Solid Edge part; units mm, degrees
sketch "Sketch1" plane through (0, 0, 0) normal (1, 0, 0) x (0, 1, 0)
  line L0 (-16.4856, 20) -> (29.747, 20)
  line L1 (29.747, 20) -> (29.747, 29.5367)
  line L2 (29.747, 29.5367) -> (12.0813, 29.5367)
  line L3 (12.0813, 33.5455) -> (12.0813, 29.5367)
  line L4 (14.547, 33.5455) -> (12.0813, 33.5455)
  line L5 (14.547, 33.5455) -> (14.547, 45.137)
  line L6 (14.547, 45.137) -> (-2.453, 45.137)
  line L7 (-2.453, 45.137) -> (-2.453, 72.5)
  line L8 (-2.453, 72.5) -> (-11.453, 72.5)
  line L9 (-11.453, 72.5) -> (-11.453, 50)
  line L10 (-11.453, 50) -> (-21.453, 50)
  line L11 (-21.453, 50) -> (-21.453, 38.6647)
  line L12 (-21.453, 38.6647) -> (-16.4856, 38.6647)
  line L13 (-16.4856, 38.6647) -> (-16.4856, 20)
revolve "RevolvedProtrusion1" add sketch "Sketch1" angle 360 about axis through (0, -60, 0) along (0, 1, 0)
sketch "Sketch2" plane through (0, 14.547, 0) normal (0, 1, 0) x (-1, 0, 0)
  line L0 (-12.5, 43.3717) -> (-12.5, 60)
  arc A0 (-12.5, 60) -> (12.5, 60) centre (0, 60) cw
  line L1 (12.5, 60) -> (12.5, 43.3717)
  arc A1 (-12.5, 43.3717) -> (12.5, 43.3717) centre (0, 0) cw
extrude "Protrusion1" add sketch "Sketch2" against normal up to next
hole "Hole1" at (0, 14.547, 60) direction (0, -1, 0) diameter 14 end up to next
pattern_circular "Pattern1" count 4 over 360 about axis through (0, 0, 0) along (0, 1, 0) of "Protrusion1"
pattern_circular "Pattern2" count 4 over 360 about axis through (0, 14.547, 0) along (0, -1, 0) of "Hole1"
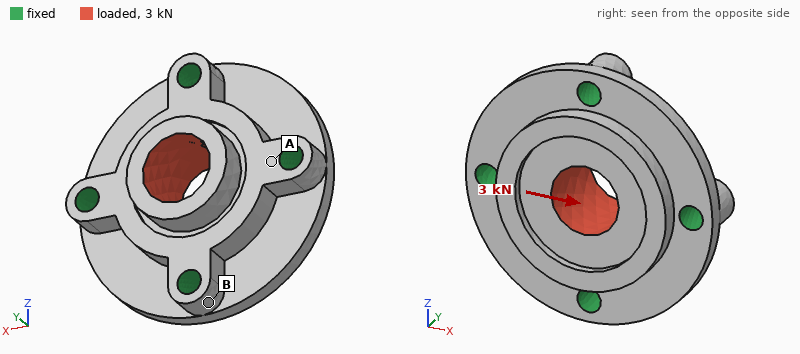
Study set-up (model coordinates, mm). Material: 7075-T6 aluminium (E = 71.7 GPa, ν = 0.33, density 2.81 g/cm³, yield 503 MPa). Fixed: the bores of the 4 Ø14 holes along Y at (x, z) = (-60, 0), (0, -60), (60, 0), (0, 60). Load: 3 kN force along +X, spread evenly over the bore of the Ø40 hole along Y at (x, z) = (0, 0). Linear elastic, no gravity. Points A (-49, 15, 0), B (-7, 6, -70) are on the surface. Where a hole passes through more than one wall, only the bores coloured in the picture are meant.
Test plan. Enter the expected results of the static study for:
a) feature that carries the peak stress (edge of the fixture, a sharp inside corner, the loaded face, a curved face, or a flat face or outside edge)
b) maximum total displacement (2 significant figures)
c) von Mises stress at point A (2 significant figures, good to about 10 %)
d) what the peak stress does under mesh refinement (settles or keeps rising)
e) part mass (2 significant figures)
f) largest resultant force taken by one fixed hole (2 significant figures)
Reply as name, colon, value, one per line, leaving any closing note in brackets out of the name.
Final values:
feature that carries the peak stress: edge of the fixture
maximum total displacement: 1.8 µm
von Mises stress at point A: 1.2 MPa
what the peak stress does under mesh refinement: keeps rising
part mass: 900 g
largest resultant force taken by one fixed hole: 1.0 kN
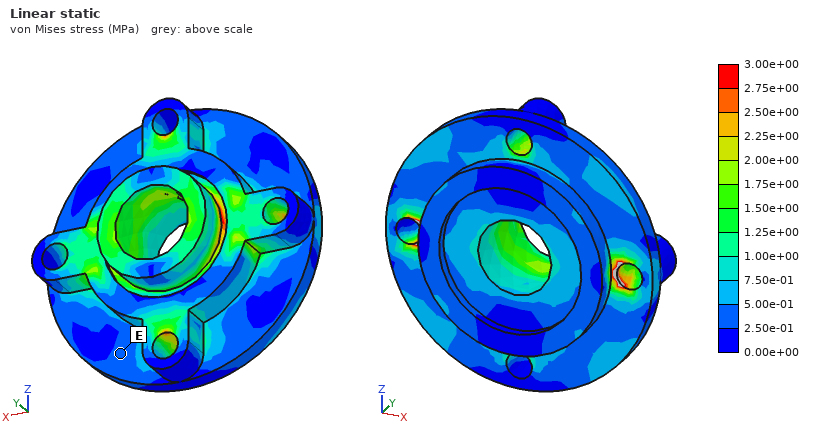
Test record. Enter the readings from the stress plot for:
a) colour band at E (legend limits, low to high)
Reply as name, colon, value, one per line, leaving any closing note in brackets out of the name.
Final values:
colour band at E: 2.50e-01 to 5.00e-01 MPa
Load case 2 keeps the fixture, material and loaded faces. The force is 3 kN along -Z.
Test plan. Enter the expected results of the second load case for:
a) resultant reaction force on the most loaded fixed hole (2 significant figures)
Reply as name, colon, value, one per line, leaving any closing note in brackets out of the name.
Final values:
resultant reaction force on the most loaded fixed hole: 1.0 kN
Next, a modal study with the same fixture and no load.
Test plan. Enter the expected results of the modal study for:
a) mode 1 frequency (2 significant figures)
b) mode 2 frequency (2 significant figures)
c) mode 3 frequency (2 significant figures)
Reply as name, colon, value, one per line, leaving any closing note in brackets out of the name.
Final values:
mode 1 frequency: 8900 Hz
mode 2 frequency: 9300 Hz
mode 3 frequency: 9300 Hz
